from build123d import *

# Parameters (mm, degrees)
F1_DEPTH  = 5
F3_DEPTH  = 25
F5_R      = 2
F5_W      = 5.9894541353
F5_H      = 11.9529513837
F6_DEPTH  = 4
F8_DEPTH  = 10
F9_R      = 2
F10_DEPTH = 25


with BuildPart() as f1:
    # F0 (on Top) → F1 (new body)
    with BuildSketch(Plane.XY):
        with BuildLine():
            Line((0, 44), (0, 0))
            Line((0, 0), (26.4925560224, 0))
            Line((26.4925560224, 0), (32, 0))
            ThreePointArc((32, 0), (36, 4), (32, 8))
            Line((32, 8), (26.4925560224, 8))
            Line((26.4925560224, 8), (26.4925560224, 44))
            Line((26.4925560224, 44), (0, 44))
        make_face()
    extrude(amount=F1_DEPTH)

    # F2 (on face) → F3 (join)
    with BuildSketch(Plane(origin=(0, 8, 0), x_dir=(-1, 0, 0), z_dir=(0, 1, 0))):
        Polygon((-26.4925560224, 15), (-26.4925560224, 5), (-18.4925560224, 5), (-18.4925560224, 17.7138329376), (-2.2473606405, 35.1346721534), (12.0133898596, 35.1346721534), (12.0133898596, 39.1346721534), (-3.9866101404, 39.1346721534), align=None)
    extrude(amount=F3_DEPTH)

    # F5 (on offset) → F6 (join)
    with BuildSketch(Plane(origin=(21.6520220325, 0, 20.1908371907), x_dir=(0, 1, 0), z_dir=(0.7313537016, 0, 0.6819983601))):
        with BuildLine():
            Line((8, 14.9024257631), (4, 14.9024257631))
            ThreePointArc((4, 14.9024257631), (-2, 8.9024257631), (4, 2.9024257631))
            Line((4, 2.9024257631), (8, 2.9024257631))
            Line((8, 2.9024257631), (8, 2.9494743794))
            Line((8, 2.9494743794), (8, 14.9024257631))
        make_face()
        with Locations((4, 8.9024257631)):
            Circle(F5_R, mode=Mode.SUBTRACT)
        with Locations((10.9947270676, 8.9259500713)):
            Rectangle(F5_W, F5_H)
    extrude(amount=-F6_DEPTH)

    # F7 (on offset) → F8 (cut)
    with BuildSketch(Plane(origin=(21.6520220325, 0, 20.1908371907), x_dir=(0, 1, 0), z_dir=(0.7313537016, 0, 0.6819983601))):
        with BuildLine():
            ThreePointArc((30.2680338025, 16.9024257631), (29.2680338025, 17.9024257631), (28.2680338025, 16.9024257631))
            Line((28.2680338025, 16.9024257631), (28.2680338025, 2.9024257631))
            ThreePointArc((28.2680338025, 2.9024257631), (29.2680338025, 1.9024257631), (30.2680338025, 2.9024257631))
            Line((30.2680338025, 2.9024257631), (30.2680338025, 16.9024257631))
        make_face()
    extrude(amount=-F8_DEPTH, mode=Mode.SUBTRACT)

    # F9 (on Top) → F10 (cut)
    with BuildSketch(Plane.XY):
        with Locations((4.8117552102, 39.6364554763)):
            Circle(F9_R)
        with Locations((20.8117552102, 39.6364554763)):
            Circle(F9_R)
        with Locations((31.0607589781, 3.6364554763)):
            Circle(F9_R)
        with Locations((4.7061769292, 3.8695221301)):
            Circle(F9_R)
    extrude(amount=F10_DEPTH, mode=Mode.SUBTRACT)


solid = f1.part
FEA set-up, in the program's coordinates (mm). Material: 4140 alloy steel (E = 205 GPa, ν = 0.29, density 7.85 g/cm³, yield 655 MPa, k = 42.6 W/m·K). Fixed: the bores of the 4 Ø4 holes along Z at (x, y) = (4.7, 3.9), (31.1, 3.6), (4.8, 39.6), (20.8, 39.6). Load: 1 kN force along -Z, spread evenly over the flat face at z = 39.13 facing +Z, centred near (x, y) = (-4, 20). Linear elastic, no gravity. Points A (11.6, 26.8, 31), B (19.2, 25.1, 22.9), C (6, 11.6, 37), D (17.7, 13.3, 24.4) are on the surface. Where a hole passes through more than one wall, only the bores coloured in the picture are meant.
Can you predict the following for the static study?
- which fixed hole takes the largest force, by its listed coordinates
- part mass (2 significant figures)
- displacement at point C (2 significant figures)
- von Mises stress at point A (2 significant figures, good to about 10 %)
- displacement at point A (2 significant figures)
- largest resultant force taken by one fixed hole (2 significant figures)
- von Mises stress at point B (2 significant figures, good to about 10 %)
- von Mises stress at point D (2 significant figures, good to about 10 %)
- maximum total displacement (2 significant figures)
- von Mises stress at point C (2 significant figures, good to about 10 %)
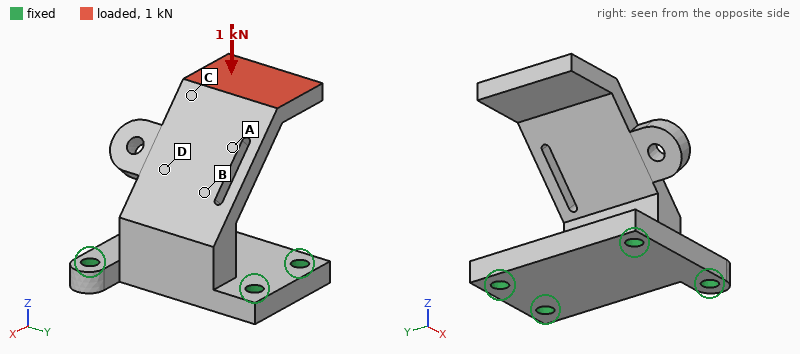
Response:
(4.7, 3.9)
100 g
0.32 mm
220 MPa
0.18 mm
860 N
320 MPa
270 MPa
0.61 mm
120 MPa
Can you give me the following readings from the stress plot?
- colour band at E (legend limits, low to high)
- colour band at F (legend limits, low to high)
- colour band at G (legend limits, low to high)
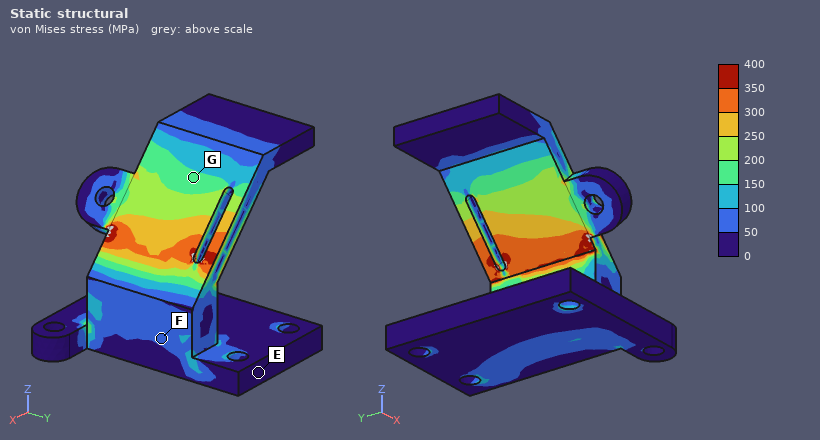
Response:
0 to 50 MPa
50 to 100 MPa
150 to 200 MPa
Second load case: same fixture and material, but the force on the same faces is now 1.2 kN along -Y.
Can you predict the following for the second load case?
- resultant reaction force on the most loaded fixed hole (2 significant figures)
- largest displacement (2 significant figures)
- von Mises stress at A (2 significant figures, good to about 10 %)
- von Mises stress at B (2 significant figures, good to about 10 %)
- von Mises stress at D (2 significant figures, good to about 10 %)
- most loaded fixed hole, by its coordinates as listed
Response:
1.8 kN
0.15 mm
38 MPa
51 MPa
52 MPa
(20.8, 39.6)
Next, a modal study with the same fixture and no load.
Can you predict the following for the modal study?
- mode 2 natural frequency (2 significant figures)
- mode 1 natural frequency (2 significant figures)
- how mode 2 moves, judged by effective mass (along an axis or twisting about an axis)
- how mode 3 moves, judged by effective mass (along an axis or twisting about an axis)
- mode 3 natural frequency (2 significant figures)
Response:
3700 Hz
1600 Hz
along Y
along X
5600 Hz
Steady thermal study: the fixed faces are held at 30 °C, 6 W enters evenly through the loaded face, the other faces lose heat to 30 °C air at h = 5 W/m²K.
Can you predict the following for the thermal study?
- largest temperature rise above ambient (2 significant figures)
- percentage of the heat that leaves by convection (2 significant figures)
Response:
63 K
9.9 %
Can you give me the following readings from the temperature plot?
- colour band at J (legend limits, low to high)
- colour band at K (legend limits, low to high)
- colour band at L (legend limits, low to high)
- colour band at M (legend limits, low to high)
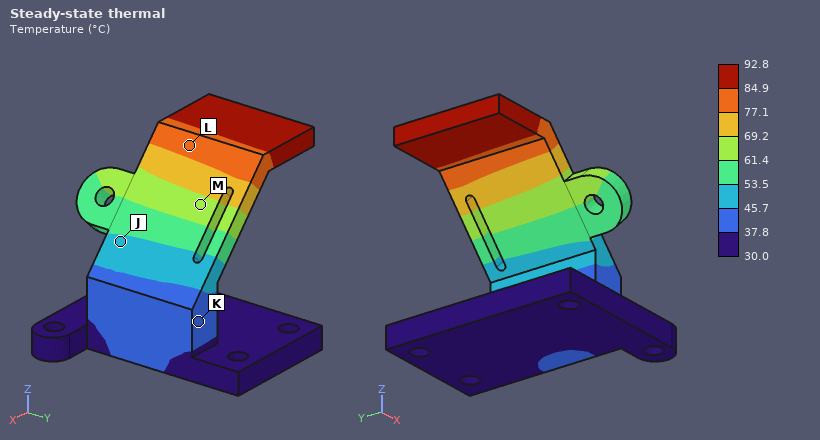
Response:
45.7 to 53.5 °C
37.8 to 45.7 °C
77.1 to 84.9 °C
61.4 to 69.2 °C
